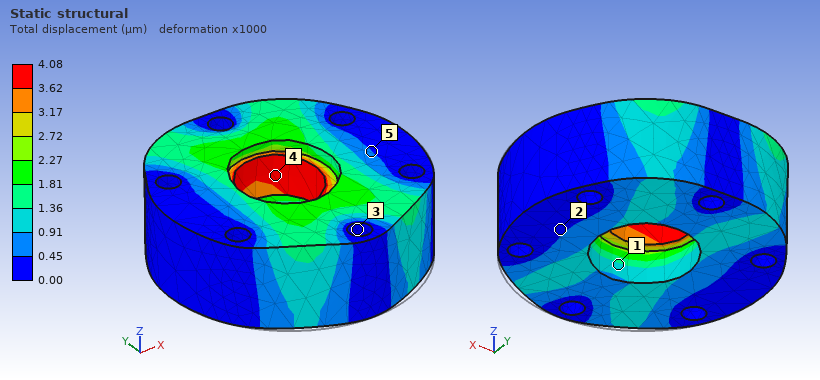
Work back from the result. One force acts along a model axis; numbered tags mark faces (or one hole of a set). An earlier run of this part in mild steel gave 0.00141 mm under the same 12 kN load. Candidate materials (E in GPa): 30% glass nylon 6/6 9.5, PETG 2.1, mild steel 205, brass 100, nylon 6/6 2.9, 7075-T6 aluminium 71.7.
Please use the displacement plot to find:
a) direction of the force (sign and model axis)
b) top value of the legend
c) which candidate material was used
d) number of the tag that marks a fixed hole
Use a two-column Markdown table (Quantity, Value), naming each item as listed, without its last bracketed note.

| Quantity | Value |
|---|---|
| direction of the force | +Y |
| top value of the legend | 4.08 µm |
| which candidate material was used | 7075-T6 aluminium |
| number of the tag that marks a fixed hole | 3 |
